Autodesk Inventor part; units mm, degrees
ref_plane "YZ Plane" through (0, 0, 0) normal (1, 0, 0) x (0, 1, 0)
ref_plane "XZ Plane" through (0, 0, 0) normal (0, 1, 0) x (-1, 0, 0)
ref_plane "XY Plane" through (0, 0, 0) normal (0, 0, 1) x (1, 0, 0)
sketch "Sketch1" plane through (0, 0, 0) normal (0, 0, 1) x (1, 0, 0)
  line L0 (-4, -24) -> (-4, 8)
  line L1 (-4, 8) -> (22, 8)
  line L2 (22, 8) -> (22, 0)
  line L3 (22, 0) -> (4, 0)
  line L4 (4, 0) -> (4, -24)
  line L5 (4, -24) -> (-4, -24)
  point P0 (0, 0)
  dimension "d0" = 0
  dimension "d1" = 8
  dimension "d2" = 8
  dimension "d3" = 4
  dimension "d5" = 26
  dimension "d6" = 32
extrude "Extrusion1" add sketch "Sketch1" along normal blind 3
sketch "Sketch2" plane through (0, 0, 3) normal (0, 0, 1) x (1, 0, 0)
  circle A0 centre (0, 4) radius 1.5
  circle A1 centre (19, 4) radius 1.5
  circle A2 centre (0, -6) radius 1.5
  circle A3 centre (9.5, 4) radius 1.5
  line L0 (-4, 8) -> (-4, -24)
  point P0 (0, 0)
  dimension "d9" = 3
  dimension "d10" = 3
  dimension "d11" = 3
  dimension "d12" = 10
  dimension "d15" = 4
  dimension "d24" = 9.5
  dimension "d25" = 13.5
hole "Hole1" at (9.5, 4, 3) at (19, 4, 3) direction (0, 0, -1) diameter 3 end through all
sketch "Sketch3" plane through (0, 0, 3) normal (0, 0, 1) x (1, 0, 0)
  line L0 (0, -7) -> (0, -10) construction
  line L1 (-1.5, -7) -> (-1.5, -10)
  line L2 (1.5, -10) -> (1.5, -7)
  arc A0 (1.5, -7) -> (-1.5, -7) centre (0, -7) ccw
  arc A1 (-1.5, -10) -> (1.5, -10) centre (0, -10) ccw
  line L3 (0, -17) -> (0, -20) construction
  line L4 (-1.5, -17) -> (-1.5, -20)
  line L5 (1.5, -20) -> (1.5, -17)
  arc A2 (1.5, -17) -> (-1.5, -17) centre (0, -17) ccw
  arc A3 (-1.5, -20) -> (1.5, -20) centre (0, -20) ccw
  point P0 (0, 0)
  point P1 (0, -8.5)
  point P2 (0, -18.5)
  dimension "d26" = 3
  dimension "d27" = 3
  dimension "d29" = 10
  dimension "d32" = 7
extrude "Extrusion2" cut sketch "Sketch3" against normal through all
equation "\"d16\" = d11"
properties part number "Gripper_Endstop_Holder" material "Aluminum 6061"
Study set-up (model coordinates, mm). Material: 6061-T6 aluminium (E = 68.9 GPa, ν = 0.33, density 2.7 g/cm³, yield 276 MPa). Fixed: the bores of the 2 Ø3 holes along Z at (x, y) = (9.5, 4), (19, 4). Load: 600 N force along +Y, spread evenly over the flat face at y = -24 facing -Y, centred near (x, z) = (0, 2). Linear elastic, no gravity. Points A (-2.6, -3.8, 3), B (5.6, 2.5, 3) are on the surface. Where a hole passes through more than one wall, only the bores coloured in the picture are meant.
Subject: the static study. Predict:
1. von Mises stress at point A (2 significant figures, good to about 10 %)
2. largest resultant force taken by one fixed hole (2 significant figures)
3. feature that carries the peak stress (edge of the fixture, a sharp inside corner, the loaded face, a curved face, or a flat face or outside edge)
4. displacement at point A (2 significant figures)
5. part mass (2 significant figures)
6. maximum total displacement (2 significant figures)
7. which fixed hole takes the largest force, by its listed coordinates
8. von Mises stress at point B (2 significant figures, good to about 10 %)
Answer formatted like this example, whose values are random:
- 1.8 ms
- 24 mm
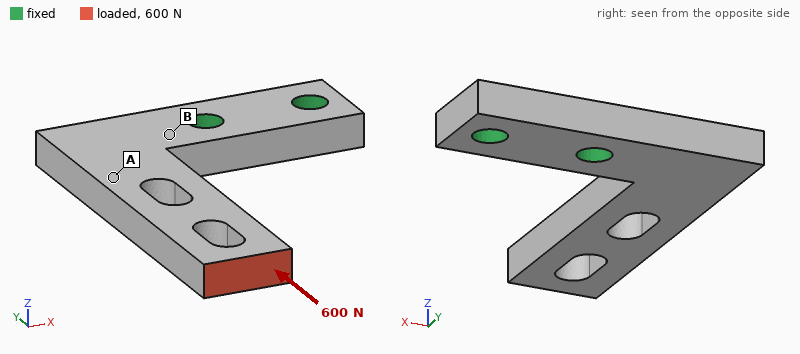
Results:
- 32 MPa
- 810 N
- edge of the fixture
- 0.062 mm
- 2.9 g
- 0.14 mm
- (9.5, 4)
- 69 MPa
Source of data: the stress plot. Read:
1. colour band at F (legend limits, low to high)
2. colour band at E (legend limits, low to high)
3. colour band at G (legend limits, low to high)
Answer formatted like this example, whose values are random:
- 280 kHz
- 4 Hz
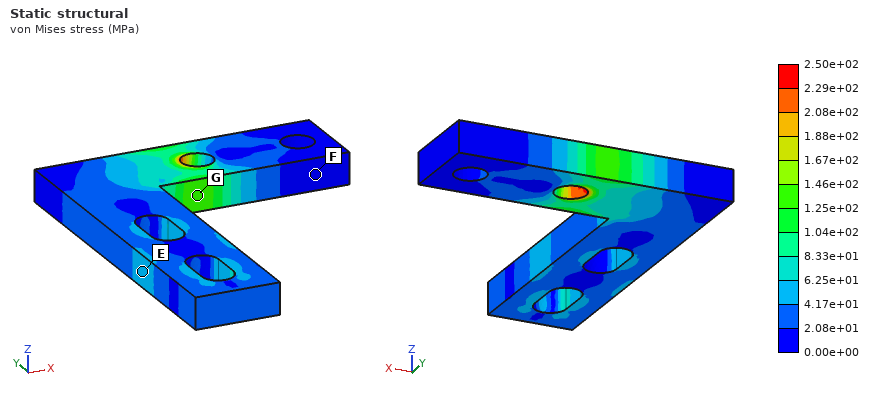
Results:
- 0.00e+00 to 2.08e+01 MPa
- 4.17e+01 to 6.25e+01 MPa
- 1.25e+02 to 1.46e+02 MPa
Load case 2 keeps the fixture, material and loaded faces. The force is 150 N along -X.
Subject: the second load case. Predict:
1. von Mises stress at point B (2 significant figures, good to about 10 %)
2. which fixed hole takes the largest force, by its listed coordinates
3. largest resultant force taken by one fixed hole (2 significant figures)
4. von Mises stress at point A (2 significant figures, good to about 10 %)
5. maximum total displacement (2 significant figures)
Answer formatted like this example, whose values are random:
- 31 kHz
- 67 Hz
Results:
- 46 MPa
- (9.5, 4)
- 220 N
- 57 MPa
- 0.28 mm
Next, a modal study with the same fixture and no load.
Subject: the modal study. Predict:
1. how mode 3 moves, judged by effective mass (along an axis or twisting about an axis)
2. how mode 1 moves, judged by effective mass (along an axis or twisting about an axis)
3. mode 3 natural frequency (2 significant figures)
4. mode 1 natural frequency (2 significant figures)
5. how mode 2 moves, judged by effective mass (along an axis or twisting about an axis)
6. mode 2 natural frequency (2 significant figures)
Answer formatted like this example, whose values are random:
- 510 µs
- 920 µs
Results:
- along Z
- along Z
- 9500 Hz
- 2600 Hz
- along X
- 5600 Hz
